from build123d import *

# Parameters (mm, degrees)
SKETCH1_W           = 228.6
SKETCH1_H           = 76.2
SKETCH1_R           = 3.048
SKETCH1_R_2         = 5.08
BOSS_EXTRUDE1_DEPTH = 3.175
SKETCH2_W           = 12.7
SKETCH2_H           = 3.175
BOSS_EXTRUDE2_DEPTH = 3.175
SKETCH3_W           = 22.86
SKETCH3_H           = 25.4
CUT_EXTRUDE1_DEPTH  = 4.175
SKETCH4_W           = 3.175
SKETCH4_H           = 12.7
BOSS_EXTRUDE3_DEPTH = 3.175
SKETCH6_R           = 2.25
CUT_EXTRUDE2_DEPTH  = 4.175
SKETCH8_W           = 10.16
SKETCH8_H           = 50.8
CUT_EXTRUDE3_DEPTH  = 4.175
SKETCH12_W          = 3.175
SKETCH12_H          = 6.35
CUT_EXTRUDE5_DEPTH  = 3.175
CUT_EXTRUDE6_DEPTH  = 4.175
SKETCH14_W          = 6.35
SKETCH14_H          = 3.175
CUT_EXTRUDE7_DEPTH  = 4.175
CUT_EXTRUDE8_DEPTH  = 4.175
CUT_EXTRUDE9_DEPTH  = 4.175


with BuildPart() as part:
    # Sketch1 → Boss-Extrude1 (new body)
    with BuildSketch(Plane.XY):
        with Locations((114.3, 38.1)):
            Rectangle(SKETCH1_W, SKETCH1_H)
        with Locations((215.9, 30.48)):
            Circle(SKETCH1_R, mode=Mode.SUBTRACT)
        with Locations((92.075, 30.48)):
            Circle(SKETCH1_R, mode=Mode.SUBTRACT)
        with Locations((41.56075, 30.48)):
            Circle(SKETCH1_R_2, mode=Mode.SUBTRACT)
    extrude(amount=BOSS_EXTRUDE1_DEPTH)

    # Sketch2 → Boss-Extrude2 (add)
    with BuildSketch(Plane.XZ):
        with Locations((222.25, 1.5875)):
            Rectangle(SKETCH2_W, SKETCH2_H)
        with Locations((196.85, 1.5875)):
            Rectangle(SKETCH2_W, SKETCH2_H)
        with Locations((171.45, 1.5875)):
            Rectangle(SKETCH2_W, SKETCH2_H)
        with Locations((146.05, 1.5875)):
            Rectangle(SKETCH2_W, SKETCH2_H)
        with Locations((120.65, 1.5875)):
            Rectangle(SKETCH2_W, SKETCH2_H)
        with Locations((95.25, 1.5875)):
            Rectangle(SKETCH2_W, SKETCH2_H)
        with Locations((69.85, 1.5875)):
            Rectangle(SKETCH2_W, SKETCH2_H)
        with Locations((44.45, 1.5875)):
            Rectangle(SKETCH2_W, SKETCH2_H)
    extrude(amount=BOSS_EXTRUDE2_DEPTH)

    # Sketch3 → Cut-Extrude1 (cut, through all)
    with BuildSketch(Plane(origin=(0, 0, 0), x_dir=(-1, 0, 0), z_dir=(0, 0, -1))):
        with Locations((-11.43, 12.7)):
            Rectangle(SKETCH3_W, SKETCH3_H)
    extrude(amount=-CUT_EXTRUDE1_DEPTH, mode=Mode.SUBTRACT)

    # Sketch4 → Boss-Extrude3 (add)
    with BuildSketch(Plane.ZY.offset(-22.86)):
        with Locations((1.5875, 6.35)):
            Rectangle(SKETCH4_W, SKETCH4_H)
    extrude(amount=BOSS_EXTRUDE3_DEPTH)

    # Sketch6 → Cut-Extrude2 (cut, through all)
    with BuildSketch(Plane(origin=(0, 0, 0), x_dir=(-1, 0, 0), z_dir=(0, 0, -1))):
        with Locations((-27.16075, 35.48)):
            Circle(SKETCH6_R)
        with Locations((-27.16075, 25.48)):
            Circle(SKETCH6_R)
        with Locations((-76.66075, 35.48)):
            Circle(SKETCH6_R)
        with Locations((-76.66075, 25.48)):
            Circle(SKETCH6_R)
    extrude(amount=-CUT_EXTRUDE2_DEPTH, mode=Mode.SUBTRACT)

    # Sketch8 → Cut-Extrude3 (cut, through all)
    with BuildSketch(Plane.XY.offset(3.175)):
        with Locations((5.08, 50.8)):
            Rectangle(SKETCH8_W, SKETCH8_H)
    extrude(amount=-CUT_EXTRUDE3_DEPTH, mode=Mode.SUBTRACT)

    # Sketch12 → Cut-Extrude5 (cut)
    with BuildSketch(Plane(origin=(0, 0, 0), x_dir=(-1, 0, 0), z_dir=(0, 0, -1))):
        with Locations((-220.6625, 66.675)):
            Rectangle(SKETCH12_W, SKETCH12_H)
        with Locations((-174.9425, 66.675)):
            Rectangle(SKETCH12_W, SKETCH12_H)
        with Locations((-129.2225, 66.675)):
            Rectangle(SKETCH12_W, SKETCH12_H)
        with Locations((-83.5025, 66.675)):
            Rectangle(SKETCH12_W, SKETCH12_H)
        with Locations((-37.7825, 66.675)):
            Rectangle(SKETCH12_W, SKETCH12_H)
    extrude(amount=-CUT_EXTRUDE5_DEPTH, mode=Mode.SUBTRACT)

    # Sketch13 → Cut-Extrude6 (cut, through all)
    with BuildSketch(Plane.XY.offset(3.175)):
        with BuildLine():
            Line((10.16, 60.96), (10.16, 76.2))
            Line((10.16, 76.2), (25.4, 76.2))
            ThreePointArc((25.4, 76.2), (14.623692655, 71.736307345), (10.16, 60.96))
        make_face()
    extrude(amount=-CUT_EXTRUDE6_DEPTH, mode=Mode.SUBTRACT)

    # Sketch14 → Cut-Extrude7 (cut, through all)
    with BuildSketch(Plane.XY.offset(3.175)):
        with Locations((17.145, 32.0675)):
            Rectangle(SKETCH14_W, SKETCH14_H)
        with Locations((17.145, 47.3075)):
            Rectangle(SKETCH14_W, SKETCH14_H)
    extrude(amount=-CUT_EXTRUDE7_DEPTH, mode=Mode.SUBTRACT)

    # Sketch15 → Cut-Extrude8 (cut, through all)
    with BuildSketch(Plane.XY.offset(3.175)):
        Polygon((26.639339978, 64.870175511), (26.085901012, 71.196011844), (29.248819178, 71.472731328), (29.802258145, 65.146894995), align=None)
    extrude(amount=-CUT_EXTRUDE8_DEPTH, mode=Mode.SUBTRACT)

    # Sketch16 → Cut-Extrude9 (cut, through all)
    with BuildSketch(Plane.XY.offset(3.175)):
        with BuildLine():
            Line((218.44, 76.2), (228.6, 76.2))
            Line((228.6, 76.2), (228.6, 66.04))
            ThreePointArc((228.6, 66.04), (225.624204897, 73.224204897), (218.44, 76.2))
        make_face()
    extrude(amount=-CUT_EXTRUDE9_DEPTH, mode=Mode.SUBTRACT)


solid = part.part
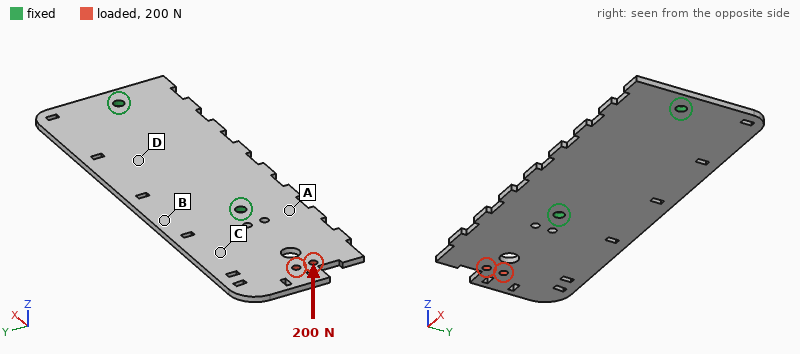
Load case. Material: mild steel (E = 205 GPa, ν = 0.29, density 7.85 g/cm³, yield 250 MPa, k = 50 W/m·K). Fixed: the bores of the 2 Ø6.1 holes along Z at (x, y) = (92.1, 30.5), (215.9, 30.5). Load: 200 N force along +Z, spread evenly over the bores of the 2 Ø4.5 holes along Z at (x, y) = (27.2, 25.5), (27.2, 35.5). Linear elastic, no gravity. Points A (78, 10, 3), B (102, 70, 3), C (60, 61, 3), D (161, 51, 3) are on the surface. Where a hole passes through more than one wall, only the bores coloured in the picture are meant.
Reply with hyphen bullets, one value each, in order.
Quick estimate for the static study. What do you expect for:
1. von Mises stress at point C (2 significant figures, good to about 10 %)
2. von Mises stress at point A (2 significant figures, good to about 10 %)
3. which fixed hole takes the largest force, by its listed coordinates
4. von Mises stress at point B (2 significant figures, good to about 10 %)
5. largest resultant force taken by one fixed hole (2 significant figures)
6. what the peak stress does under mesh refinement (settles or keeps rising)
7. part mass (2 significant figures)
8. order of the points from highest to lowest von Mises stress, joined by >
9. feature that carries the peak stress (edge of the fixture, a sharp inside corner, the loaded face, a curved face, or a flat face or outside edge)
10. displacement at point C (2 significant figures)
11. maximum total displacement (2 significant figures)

- 49 MPa
- 85 MPa
- (92.1, 30.5)
- 31 MPa
- 220 N
- keeps rising
- 400 g
- A > C > B > D
- edge of the fixture
- 0.18 mm
- 0.76 mm
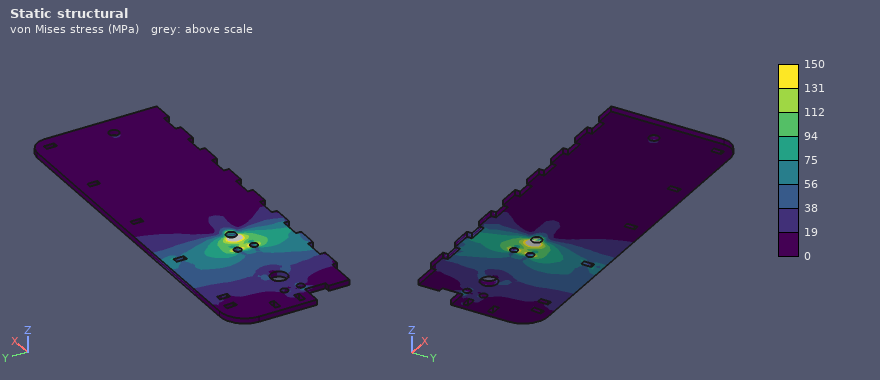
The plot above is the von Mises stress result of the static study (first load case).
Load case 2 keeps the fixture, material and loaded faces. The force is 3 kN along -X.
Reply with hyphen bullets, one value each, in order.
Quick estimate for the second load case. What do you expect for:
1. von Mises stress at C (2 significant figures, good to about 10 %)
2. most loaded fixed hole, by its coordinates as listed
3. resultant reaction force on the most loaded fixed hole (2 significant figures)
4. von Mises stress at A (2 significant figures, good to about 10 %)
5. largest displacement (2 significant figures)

- 8.0 MPa
- (92.1, 30.5)
- 2.5 kN
- 12 MPa
- 14 µm
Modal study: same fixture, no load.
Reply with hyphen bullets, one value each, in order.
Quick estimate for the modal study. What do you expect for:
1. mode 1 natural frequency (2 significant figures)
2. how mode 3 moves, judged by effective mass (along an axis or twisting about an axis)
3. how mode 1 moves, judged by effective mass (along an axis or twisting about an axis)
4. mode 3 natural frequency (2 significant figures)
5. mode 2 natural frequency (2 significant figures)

- 390 Hz
- along Z
- along Z
- 870 Hz
- 720 Hz
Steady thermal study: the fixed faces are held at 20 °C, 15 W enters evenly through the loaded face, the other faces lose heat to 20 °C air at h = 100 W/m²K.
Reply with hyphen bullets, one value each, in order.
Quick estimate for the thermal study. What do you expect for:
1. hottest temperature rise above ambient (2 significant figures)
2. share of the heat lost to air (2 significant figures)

- 48 K
- 94 %
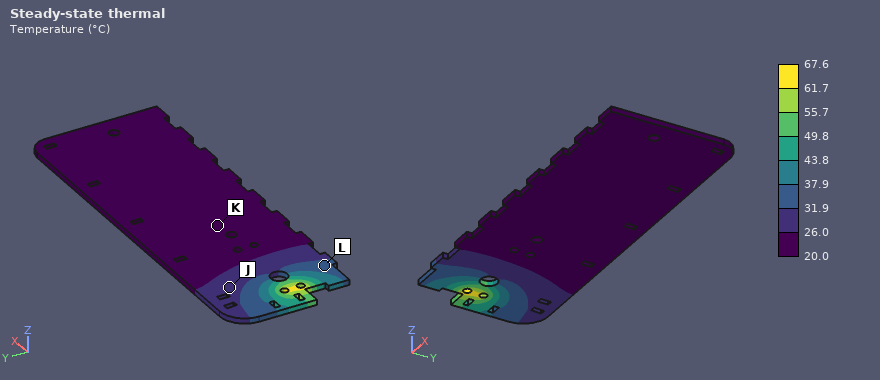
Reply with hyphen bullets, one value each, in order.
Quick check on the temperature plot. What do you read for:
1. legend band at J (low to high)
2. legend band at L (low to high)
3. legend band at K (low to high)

- 26.0 to 31.9 °C
- 31.9 to 37.9 °C
- 20.0 to 26.0 °C
